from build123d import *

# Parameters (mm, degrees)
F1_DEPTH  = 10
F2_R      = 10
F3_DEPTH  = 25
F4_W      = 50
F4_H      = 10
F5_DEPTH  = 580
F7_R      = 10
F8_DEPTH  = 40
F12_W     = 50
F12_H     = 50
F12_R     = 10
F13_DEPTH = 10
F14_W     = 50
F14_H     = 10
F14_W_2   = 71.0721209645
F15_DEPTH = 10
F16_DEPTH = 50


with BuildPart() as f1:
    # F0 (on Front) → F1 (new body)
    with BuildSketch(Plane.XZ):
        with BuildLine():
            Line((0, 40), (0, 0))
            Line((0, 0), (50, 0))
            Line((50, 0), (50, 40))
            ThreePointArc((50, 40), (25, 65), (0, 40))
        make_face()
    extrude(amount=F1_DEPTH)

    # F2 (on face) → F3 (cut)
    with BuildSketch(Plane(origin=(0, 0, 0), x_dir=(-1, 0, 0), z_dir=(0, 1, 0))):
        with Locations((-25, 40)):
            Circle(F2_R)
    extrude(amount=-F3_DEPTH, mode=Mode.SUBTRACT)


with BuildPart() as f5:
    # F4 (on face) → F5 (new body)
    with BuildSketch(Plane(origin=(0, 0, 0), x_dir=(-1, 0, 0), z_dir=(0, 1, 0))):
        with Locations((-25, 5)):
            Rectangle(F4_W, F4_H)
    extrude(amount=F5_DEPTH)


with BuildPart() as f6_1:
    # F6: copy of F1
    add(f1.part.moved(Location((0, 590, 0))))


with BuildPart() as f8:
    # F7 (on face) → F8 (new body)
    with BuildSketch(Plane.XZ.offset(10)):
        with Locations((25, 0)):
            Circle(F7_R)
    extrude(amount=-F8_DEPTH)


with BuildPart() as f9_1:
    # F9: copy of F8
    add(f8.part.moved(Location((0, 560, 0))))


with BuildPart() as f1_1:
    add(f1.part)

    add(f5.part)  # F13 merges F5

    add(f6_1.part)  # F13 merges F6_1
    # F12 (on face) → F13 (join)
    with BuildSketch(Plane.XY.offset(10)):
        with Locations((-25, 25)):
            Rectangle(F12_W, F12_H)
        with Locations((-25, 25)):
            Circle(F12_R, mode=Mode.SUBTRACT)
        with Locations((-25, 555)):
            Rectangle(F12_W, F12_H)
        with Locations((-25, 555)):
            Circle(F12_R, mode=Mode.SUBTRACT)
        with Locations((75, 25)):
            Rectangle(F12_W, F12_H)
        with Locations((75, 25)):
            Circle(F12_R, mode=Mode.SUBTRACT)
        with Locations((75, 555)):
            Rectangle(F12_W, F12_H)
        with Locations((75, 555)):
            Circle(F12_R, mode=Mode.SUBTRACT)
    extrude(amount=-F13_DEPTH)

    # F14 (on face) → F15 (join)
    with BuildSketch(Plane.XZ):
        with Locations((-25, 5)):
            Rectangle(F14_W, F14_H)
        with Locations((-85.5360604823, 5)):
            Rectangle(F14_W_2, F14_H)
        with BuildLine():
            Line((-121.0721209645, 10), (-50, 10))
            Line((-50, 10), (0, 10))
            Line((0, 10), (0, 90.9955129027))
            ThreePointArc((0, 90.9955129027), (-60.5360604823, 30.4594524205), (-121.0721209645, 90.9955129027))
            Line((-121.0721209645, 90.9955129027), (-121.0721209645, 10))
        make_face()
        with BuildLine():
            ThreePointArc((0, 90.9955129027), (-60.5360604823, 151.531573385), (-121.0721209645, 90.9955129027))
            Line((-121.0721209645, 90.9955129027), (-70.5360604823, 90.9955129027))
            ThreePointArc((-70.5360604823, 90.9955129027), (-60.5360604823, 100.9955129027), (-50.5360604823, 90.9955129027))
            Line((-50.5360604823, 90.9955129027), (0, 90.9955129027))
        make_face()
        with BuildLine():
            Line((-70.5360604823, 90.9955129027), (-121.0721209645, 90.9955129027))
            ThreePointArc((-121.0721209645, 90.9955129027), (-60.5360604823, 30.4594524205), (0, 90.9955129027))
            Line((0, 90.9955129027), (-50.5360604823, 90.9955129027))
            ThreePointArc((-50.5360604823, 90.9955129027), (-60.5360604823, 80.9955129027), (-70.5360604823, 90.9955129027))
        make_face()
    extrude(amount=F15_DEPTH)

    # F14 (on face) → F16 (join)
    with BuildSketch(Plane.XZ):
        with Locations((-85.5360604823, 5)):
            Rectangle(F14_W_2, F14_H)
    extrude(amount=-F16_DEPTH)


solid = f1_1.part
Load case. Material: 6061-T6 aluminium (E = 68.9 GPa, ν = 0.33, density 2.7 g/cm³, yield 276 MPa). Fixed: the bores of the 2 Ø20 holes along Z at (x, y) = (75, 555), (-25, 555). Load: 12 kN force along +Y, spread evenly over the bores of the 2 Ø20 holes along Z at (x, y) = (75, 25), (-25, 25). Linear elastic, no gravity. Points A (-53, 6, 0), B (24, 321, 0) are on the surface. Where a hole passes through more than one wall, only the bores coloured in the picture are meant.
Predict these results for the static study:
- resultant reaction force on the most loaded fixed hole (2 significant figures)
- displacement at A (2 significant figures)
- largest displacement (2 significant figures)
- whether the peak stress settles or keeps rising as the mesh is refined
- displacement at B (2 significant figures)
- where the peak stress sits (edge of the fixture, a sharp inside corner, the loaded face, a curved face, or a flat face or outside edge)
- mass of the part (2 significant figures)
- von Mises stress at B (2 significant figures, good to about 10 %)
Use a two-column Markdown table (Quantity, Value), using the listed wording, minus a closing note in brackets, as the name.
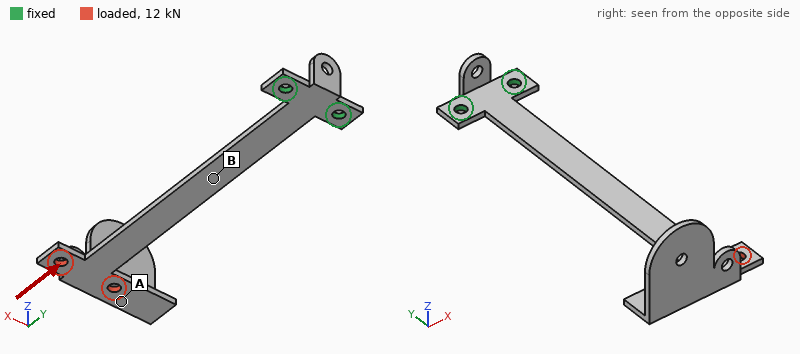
| Quantity | Value |
|---|---|
| resultant reaction force on the most loaded fixed hole | 6.1 kN |
| displacement at A | 0.23 mm |
| largest displacement | 0.26 mm |
| whether the peak stress settles or keeps rising as the mesh is refined | keeps rising |
| displacement at B | 0.092 mm |
| where the peak stress sits | a sharp inside corner |
| mass of the part | 1.7 kg |
| von Mises stress at B | 24 MPa |
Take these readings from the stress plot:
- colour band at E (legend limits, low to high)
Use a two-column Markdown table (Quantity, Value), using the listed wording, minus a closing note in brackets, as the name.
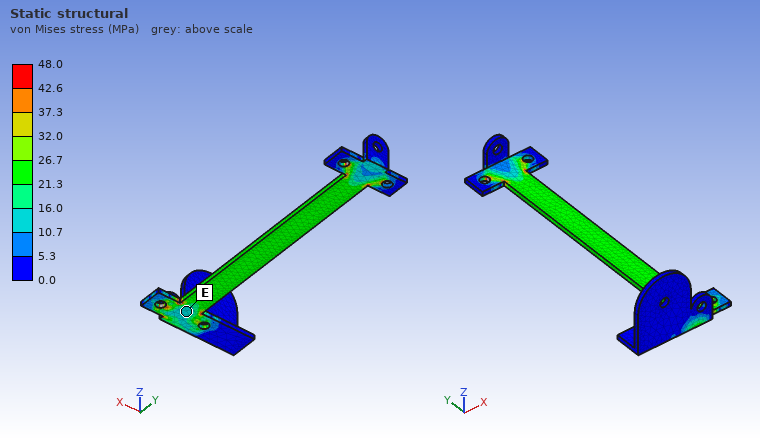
| Quantity | Value |
|---|---|
| colour band at E | 10.7 to 16.0 MPa |
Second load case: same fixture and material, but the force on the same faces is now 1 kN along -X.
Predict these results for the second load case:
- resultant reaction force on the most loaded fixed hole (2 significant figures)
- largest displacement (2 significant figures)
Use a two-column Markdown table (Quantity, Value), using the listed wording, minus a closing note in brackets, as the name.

| Quantity | Value |
|---|---|
| resultant reaction force on the most loaded fixed hole | 6.3 kN |
| largest displacement | 7.8 mm |
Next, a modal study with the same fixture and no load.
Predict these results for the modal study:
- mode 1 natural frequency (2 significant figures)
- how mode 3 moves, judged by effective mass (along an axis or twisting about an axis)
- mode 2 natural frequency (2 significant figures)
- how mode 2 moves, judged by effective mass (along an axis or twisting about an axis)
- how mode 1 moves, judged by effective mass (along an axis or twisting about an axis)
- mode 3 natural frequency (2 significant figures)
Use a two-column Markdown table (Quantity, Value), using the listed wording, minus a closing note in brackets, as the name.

| Quantity | Value |
|---|---|
| mode 1 natural frequency | 12 Hz |
| how mode 3 moves, judged by effective mass | along X |
| mode 2 natural frequency | 49 Hz |
| how mode 2 moves, judged by effective mass | along X |
| how mode 1 moves, judged by effective mass | along Z |
| mode 3 natural frequency | 77 Hz |
